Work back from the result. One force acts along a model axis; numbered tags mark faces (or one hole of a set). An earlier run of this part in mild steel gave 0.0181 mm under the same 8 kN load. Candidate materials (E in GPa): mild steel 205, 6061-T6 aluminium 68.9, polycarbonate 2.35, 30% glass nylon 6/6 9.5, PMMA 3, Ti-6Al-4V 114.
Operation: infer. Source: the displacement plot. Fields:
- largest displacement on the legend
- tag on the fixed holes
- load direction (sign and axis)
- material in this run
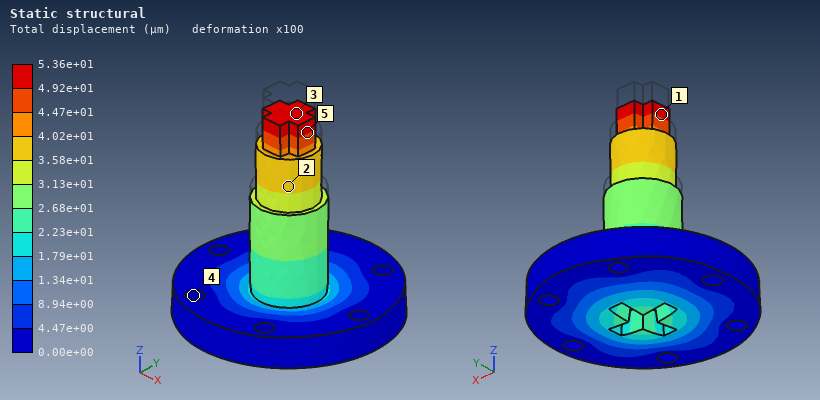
5.36e+01 µm
4
-Z
6061-T6 aluminium
